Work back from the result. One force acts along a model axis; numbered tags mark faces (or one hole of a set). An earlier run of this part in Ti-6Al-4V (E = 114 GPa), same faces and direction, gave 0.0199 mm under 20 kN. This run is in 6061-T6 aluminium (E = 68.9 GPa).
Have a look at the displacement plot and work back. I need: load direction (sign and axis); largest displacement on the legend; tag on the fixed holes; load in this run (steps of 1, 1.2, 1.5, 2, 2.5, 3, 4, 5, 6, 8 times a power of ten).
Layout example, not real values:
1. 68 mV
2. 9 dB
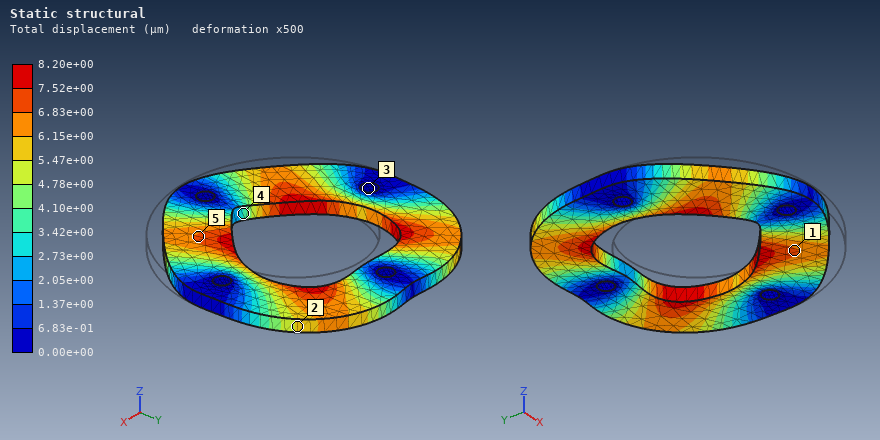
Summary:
1. +Y
2. 8.20e+00 µm
3. 3
4. 5 kN
